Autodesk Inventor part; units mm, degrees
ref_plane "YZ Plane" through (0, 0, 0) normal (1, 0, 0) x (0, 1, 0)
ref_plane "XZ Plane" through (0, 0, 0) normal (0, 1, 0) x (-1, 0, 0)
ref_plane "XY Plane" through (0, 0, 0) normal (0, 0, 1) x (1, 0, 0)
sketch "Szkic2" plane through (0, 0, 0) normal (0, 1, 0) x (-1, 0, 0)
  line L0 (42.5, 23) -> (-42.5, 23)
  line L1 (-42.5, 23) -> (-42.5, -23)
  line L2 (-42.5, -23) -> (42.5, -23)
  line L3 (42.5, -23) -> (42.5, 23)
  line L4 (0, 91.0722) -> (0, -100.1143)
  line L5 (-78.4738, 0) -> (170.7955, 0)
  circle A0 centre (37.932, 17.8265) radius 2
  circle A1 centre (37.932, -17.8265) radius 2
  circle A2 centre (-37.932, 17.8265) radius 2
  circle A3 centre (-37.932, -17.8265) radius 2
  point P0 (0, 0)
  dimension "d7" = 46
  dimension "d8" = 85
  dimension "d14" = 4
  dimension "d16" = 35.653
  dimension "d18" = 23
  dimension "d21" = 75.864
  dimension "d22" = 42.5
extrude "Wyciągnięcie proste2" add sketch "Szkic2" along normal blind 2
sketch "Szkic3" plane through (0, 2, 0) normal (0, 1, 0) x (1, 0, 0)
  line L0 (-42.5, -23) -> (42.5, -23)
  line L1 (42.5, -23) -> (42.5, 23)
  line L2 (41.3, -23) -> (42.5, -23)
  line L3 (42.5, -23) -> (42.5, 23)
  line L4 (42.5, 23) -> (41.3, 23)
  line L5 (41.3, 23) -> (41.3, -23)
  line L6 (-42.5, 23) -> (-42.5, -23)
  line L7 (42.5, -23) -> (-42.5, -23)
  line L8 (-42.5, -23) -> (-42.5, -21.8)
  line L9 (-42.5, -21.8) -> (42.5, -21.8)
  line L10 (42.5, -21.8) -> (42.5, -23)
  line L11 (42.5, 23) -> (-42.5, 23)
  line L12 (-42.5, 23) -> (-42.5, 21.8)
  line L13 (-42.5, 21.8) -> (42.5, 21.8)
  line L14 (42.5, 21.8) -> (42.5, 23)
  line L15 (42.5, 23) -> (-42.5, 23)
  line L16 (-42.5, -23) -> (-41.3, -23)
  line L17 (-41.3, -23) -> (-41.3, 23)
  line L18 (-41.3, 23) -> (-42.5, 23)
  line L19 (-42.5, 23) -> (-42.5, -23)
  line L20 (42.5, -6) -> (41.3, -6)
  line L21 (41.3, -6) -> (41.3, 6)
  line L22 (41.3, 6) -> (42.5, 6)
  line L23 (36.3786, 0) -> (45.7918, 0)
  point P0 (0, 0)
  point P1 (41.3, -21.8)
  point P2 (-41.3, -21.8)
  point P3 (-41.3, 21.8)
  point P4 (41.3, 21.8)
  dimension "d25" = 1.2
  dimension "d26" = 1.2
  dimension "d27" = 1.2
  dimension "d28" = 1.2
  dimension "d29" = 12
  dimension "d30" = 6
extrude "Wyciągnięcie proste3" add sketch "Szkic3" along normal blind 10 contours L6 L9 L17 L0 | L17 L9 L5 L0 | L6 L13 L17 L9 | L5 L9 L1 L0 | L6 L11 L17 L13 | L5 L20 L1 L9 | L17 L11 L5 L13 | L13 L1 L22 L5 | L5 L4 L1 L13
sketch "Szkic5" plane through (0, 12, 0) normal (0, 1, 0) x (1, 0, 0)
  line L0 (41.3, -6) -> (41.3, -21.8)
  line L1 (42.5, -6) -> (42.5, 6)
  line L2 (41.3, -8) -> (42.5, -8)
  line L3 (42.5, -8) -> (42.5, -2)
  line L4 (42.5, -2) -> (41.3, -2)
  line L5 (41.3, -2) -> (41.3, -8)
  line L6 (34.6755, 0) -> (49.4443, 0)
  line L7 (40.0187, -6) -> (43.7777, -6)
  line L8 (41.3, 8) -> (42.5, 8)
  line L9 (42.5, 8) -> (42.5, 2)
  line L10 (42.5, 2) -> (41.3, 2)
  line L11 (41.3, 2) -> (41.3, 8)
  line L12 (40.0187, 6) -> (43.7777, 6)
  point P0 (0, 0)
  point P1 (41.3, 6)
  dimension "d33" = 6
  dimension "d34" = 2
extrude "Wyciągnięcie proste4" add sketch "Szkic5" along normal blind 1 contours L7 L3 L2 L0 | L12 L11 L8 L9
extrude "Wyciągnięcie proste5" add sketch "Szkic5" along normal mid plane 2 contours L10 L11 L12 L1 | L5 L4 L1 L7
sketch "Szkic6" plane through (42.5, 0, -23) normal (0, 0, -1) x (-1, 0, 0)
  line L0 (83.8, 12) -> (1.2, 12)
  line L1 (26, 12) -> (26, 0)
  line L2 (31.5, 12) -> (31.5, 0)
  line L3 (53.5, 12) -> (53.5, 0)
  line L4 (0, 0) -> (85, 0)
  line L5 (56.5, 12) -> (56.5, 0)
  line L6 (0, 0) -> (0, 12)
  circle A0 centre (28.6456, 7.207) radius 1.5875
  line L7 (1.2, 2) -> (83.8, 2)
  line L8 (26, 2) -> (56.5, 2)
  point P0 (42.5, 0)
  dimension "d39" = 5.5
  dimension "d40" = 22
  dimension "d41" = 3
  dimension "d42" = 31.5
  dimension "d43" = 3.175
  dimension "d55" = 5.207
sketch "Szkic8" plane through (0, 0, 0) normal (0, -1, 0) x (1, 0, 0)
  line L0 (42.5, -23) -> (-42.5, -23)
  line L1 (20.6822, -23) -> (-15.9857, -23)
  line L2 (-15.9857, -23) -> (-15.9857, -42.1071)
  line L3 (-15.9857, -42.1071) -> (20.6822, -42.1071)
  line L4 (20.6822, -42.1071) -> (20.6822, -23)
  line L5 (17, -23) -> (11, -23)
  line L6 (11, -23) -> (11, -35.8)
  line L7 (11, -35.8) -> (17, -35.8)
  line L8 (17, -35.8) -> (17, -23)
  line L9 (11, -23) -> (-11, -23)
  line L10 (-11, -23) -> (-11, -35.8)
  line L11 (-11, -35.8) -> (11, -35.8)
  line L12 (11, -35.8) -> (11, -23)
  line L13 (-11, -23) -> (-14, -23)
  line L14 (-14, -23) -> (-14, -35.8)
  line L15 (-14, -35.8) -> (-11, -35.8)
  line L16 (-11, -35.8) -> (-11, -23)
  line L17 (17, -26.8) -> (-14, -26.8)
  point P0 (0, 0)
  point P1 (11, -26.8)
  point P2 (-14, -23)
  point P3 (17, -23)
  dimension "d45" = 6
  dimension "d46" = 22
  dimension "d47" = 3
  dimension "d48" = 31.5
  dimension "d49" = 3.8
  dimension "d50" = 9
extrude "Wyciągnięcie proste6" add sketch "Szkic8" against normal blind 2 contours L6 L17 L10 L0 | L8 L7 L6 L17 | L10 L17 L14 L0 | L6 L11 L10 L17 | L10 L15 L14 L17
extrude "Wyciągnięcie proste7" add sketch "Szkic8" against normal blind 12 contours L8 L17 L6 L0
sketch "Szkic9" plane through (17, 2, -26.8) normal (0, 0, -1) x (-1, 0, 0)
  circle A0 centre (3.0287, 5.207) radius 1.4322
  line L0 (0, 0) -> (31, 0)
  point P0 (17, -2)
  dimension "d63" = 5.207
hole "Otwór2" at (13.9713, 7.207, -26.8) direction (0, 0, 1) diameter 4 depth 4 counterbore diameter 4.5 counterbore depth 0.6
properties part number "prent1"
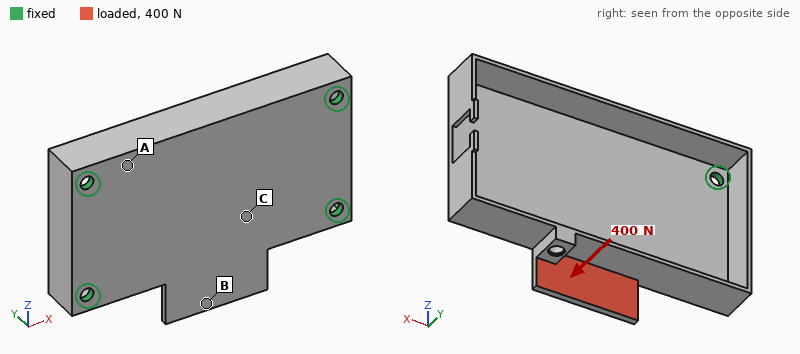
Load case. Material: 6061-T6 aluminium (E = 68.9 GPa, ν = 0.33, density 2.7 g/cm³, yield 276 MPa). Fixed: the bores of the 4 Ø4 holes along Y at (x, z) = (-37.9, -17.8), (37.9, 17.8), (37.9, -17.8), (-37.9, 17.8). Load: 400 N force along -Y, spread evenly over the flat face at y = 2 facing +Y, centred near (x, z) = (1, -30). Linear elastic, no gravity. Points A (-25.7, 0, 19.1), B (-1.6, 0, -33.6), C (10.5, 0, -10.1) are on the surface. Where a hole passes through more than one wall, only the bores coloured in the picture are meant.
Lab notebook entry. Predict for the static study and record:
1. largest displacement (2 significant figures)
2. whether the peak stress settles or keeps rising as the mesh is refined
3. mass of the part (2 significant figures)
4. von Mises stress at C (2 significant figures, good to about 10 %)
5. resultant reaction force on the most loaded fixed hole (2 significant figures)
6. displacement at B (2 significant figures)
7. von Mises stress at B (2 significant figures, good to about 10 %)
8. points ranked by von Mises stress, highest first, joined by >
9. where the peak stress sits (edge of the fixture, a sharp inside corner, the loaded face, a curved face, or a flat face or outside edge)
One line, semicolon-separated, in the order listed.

0.42 mm; keeps rising; 31 g; 44 MPa; 420 N; 0.37 mm; 29 MPa; C > B > A; edge of the fixture
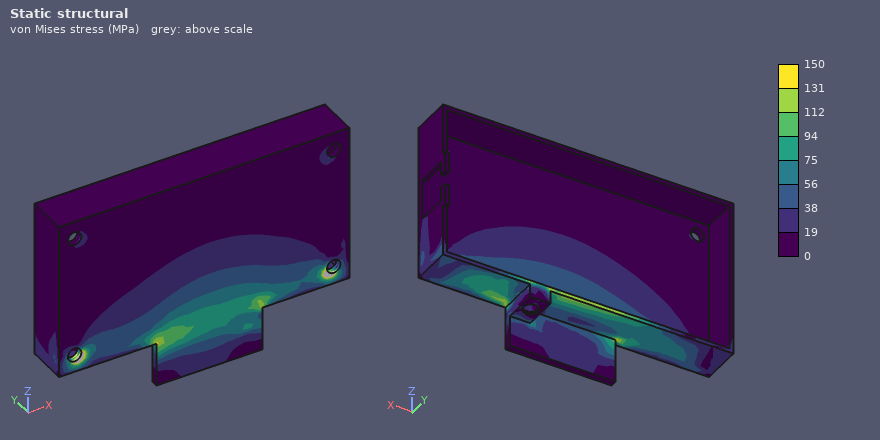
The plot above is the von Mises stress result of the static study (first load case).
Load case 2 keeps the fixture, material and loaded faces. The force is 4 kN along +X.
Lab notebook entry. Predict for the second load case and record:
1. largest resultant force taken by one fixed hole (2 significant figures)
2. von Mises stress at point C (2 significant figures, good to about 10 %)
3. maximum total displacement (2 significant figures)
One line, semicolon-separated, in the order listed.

1.6 kN; 26 MPa; 0.12 mm
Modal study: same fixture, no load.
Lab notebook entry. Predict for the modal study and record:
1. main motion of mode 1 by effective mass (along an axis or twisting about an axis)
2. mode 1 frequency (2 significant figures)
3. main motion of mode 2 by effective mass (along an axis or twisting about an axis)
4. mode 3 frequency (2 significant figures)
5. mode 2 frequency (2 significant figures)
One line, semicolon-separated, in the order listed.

along Y; 3000 Hz; along Y; 5800 Hz; 3500 Hz
